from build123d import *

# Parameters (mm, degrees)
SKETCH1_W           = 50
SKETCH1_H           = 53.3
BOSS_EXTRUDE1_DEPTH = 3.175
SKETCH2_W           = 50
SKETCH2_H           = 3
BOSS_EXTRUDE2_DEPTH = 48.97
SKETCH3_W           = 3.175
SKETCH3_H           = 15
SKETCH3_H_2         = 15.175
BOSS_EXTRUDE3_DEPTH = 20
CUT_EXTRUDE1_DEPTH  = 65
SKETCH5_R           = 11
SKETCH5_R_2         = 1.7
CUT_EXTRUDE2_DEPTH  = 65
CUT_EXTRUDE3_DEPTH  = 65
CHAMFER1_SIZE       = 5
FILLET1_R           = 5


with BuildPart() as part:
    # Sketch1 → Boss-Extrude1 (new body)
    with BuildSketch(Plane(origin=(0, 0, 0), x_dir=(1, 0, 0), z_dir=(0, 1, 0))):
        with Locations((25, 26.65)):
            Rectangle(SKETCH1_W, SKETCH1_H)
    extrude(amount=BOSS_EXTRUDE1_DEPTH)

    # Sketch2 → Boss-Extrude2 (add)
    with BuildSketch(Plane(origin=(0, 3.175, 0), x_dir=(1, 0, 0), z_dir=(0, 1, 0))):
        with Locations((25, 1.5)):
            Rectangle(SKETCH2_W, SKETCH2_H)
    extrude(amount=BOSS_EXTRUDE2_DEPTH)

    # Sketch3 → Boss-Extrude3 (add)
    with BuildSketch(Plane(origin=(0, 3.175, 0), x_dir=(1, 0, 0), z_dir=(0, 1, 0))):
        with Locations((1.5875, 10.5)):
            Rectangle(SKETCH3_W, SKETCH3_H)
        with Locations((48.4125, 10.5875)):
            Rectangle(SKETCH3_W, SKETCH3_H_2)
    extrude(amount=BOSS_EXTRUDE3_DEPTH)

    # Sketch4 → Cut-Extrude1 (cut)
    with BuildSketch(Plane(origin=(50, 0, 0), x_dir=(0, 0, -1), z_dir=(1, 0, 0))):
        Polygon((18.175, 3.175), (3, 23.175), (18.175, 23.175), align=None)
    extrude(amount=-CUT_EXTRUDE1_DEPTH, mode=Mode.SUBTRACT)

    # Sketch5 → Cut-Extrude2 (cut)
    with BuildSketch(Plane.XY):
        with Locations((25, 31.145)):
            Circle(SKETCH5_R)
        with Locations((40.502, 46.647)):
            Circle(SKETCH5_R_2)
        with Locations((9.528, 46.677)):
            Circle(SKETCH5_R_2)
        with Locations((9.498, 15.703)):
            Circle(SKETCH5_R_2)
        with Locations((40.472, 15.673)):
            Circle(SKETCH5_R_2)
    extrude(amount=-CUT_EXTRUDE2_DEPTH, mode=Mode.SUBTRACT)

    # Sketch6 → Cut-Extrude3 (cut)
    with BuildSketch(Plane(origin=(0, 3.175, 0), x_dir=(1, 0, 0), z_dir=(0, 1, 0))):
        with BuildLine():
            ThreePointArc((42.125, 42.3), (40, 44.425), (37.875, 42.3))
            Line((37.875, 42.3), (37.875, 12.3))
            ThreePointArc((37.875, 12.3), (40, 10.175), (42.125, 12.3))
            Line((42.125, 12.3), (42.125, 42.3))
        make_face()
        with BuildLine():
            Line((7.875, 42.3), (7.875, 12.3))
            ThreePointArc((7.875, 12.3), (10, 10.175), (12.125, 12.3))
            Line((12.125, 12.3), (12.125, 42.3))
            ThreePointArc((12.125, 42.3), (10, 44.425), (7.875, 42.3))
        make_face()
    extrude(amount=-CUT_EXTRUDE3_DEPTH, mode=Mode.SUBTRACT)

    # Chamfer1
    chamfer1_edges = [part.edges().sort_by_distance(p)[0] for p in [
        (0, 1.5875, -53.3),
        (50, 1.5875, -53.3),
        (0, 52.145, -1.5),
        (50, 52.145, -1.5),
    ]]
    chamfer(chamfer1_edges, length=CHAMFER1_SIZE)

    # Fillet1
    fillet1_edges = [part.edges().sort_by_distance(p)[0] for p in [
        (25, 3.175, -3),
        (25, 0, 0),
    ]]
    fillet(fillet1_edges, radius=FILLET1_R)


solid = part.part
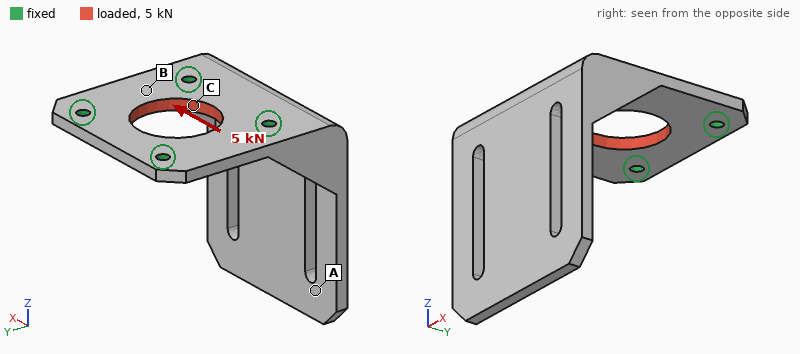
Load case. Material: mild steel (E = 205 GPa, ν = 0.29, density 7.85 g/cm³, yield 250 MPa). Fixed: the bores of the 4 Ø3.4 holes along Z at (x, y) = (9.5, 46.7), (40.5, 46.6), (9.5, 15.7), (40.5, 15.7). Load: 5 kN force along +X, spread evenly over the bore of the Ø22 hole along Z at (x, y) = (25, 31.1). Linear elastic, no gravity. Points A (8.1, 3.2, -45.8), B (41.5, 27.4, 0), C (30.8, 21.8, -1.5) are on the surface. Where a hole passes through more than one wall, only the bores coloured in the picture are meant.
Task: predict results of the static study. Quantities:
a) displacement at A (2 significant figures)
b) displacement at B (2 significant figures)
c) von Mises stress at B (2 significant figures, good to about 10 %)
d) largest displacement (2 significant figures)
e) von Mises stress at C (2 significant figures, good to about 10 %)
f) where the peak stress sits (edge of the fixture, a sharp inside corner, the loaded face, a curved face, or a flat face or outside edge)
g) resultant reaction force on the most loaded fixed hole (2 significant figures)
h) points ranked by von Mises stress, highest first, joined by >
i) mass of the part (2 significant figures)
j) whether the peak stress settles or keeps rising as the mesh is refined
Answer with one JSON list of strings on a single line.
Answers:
["1.2 µm", "3.0 µm", "22 MPa", "3.8 µm", "47 MPa", "edge of the fixture", "1.3 kN", "C > B > A", "110 g", "keeps rising"]
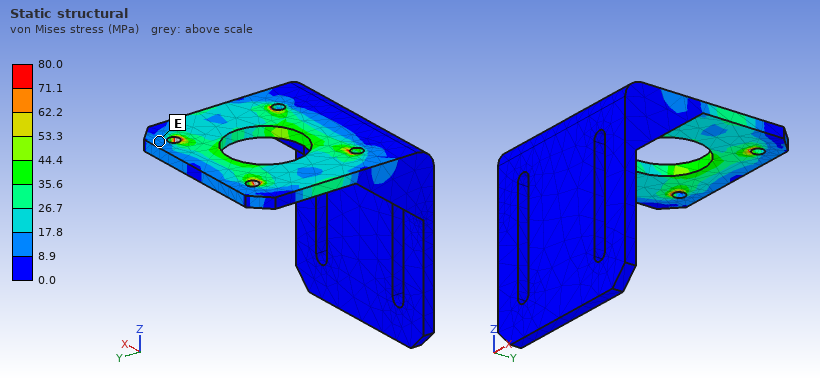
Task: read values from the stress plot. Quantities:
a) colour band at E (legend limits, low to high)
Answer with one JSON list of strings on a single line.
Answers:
["8.9 to 17.8 MPa"]
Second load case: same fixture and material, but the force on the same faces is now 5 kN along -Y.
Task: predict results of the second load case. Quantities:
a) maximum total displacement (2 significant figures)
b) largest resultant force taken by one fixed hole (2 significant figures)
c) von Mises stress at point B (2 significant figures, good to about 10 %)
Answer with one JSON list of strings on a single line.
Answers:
["5.0 µm", "1.3 kN", "22 MPa"]
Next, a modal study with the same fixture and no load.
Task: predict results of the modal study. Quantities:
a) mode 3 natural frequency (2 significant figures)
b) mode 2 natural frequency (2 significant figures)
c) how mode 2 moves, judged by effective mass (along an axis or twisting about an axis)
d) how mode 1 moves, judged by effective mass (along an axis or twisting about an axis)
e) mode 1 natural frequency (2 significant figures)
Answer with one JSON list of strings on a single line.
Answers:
["3500 Hz", "2200 Hz", "along X", "along Y", "1000 Hz"]
